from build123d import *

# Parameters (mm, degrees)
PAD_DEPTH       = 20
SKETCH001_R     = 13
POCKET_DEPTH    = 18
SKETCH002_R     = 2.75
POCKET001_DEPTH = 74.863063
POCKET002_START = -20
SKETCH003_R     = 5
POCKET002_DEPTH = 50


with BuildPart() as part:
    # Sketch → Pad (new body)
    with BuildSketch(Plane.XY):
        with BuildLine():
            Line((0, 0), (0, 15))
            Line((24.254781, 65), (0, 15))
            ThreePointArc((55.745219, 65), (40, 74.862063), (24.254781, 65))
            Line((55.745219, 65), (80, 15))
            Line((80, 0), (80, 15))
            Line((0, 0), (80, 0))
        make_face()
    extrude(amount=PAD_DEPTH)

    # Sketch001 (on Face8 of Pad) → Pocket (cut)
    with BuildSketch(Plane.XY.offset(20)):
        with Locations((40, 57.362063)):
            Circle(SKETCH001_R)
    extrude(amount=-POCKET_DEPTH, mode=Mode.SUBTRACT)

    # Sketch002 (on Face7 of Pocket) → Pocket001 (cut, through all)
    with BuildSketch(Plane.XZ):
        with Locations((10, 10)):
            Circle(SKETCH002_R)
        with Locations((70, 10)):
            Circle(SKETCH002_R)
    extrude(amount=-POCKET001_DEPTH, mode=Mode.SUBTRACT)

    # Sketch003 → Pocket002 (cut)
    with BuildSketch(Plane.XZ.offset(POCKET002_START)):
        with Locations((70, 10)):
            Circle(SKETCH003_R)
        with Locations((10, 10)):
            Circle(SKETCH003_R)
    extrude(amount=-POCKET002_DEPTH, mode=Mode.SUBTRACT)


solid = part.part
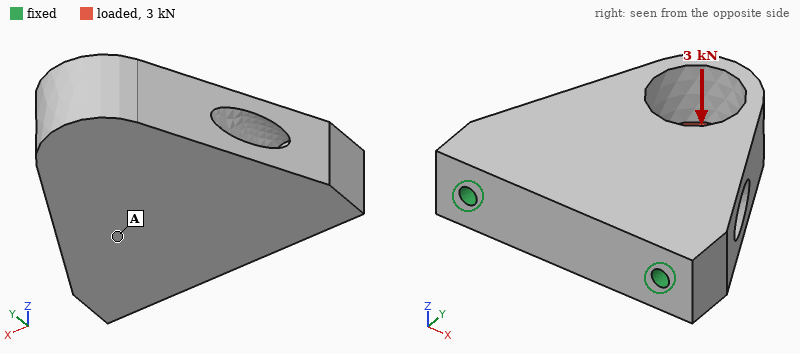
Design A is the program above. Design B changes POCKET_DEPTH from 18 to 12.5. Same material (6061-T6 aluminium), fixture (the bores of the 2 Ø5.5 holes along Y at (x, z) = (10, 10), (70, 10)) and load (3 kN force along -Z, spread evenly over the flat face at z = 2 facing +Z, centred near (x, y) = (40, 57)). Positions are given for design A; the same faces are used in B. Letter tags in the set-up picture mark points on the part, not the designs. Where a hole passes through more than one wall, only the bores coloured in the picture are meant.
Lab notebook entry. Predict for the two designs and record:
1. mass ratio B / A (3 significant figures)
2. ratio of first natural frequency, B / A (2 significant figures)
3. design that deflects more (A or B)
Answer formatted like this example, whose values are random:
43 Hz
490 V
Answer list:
1.04
0.93
A
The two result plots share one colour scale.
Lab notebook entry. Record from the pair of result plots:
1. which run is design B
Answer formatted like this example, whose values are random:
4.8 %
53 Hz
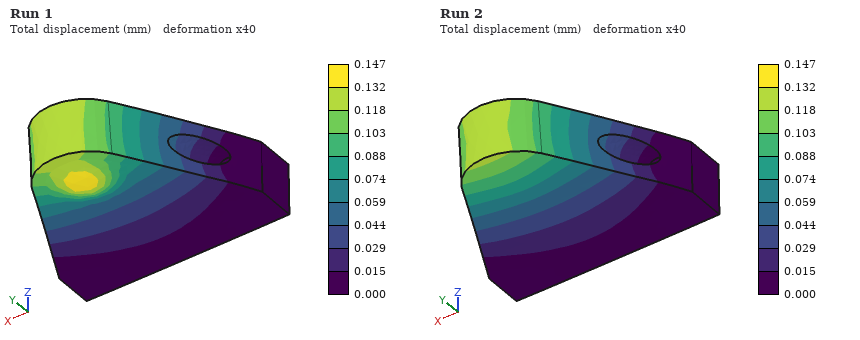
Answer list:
Run 2
